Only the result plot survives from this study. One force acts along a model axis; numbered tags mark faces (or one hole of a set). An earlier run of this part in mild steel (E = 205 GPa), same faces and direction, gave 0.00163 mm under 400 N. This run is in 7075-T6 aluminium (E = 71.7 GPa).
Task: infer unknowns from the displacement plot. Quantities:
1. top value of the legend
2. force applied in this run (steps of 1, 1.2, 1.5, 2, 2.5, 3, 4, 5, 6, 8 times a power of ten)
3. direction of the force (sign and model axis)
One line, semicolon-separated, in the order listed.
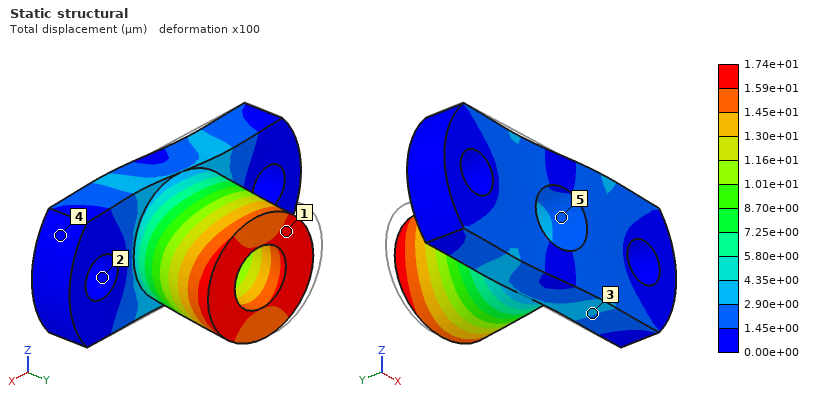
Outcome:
1.74e+01 µm; 1.5 kN; +X
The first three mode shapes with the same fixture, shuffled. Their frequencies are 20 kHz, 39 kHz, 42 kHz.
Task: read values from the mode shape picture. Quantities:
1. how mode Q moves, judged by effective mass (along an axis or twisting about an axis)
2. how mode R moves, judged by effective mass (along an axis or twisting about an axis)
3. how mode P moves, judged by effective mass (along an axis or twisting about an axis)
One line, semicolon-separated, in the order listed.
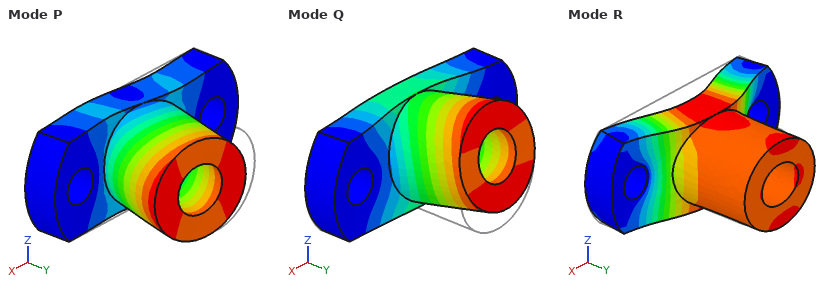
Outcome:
along Z; along Y; along X
